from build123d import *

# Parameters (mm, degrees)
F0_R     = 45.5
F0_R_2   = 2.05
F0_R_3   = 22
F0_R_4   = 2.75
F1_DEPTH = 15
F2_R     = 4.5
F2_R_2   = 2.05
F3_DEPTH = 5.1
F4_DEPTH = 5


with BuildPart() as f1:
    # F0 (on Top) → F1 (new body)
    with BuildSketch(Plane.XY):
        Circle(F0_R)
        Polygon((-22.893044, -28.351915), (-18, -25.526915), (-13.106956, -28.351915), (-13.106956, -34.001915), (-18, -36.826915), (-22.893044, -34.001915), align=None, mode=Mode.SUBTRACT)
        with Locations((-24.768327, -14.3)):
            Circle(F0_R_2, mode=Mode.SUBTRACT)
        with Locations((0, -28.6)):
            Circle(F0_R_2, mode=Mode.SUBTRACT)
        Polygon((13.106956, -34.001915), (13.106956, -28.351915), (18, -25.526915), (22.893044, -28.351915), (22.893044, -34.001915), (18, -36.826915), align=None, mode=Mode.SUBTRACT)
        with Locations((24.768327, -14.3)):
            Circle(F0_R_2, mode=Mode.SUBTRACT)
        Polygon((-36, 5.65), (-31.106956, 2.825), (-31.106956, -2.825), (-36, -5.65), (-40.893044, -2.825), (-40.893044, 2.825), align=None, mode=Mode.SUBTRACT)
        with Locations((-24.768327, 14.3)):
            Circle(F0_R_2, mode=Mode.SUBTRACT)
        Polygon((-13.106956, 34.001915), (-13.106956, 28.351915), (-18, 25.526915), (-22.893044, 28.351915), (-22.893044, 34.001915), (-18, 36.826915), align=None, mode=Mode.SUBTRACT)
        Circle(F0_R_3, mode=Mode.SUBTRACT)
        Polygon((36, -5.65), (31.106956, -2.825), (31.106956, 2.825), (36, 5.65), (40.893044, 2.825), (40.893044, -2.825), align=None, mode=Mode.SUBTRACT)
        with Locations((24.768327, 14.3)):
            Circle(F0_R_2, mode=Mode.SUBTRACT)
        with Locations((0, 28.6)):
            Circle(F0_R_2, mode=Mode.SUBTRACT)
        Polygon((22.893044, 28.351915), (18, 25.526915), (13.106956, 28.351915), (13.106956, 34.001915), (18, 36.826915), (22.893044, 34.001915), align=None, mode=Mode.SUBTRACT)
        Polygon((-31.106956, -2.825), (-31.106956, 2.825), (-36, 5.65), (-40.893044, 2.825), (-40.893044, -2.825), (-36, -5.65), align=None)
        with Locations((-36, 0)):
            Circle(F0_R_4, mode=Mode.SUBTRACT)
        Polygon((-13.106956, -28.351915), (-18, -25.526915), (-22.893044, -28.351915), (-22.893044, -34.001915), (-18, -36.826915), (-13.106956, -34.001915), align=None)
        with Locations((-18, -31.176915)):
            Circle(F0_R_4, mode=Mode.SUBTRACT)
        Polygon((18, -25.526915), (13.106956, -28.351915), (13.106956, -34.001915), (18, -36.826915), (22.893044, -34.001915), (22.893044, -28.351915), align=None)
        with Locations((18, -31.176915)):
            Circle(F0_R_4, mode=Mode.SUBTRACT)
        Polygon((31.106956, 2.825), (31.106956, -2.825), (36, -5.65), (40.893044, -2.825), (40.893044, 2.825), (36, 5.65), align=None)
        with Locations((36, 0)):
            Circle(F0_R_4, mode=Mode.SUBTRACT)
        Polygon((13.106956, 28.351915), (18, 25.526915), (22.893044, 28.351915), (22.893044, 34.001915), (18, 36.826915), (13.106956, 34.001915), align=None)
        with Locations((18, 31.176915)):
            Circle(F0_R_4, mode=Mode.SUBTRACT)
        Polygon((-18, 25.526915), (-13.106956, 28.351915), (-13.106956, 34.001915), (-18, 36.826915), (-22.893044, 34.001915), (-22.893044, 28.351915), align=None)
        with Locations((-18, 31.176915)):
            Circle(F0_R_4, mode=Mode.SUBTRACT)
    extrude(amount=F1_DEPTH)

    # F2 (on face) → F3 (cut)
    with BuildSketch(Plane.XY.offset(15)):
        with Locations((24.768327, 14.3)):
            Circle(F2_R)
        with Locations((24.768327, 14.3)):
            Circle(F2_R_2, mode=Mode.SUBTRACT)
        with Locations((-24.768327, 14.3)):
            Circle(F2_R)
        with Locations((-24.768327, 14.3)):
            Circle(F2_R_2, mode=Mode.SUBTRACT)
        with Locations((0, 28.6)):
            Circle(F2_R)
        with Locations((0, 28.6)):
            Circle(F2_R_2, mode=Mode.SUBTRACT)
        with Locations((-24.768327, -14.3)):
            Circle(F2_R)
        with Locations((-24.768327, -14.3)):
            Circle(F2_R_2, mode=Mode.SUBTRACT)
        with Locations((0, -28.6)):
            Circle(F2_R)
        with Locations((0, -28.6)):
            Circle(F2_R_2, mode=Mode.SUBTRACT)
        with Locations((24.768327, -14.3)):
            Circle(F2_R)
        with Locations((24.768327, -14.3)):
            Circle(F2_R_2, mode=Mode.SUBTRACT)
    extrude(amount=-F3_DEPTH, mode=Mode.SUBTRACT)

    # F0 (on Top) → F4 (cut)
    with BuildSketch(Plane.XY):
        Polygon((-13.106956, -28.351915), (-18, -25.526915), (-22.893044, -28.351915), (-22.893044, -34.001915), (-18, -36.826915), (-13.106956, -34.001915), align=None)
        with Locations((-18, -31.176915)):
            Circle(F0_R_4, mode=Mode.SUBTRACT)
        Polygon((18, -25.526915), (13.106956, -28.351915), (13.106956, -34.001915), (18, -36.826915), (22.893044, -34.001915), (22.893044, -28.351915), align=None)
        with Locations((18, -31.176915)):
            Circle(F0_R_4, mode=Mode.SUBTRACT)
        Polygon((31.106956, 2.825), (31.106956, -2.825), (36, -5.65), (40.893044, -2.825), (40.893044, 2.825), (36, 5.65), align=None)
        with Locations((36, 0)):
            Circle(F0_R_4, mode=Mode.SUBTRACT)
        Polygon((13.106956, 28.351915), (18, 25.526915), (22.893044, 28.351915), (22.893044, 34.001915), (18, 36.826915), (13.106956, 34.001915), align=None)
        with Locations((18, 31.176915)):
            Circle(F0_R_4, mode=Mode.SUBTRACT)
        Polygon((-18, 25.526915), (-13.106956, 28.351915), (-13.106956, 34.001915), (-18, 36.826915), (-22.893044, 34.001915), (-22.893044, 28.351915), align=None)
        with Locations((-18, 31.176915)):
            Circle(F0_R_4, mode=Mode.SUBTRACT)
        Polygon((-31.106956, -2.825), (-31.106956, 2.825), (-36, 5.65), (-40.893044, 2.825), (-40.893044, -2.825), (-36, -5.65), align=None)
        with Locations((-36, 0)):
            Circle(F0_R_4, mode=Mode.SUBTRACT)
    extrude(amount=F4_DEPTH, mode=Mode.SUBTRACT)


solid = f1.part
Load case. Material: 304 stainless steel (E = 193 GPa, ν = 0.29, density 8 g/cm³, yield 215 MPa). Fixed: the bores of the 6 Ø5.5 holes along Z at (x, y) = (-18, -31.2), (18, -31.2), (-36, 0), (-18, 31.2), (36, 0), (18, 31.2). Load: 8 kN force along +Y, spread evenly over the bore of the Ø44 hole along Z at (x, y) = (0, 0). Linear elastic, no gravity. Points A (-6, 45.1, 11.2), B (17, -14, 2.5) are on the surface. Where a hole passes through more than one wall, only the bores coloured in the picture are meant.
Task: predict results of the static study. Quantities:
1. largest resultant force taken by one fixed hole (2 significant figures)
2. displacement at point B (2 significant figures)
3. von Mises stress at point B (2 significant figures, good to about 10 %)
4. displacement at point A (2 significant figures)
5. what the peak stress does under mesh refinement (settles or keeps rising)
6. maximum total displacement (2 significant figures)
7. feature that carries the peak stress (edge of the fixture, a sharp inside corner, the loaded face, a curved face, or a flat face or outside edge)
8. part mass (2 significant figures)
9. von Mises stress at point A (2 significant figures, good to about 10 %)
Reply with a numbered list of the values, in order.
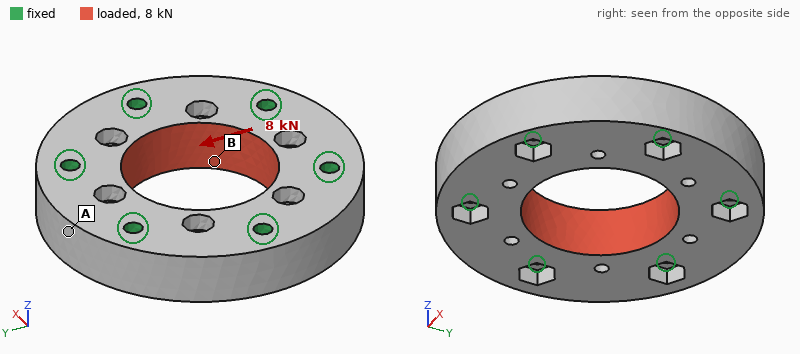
1. 1.5 kN
2. 0.73 µm
3. 6.7 MPa
4. 0.49 µm
5. keeps rising
6. 1.1 µm
7. edge of the fixture
8. 540 g
9. 3.1 MPa
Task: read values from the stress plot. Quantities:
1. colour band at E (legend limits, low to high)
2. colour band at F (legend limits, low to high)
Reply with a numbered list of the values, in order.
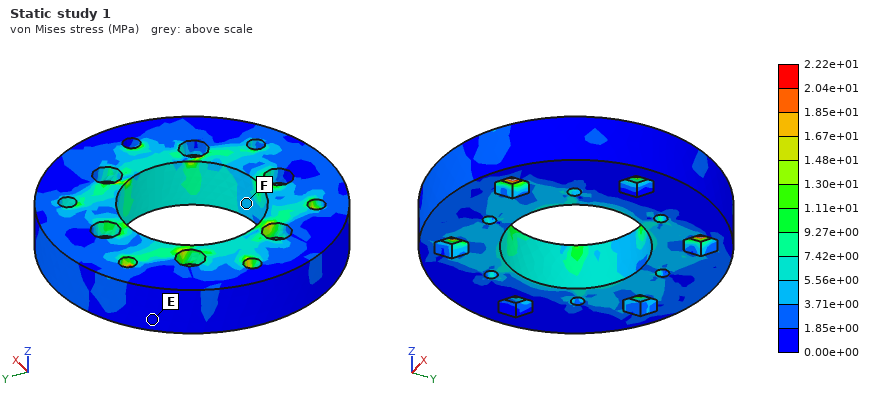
1. 0.00e+00 to 1.85e+00 MPa
2. 3.71e+00 to 5.56e+00 MPa
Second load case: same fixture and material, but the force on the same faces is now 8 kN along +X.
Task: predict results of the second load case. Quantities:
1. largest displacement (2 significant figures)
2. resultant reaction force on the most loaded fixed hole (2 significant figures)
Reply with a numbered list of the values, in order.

1. 1.0 µm
2. 1.6 kN
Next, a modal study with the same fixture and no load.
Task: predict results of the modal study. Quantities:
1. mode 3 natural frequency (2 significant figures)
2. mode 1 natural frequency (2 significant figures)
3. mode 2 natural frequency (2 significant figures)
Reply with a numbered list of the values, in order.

1. 22 kHz
2. 22 kHz
3. 22 kHz
